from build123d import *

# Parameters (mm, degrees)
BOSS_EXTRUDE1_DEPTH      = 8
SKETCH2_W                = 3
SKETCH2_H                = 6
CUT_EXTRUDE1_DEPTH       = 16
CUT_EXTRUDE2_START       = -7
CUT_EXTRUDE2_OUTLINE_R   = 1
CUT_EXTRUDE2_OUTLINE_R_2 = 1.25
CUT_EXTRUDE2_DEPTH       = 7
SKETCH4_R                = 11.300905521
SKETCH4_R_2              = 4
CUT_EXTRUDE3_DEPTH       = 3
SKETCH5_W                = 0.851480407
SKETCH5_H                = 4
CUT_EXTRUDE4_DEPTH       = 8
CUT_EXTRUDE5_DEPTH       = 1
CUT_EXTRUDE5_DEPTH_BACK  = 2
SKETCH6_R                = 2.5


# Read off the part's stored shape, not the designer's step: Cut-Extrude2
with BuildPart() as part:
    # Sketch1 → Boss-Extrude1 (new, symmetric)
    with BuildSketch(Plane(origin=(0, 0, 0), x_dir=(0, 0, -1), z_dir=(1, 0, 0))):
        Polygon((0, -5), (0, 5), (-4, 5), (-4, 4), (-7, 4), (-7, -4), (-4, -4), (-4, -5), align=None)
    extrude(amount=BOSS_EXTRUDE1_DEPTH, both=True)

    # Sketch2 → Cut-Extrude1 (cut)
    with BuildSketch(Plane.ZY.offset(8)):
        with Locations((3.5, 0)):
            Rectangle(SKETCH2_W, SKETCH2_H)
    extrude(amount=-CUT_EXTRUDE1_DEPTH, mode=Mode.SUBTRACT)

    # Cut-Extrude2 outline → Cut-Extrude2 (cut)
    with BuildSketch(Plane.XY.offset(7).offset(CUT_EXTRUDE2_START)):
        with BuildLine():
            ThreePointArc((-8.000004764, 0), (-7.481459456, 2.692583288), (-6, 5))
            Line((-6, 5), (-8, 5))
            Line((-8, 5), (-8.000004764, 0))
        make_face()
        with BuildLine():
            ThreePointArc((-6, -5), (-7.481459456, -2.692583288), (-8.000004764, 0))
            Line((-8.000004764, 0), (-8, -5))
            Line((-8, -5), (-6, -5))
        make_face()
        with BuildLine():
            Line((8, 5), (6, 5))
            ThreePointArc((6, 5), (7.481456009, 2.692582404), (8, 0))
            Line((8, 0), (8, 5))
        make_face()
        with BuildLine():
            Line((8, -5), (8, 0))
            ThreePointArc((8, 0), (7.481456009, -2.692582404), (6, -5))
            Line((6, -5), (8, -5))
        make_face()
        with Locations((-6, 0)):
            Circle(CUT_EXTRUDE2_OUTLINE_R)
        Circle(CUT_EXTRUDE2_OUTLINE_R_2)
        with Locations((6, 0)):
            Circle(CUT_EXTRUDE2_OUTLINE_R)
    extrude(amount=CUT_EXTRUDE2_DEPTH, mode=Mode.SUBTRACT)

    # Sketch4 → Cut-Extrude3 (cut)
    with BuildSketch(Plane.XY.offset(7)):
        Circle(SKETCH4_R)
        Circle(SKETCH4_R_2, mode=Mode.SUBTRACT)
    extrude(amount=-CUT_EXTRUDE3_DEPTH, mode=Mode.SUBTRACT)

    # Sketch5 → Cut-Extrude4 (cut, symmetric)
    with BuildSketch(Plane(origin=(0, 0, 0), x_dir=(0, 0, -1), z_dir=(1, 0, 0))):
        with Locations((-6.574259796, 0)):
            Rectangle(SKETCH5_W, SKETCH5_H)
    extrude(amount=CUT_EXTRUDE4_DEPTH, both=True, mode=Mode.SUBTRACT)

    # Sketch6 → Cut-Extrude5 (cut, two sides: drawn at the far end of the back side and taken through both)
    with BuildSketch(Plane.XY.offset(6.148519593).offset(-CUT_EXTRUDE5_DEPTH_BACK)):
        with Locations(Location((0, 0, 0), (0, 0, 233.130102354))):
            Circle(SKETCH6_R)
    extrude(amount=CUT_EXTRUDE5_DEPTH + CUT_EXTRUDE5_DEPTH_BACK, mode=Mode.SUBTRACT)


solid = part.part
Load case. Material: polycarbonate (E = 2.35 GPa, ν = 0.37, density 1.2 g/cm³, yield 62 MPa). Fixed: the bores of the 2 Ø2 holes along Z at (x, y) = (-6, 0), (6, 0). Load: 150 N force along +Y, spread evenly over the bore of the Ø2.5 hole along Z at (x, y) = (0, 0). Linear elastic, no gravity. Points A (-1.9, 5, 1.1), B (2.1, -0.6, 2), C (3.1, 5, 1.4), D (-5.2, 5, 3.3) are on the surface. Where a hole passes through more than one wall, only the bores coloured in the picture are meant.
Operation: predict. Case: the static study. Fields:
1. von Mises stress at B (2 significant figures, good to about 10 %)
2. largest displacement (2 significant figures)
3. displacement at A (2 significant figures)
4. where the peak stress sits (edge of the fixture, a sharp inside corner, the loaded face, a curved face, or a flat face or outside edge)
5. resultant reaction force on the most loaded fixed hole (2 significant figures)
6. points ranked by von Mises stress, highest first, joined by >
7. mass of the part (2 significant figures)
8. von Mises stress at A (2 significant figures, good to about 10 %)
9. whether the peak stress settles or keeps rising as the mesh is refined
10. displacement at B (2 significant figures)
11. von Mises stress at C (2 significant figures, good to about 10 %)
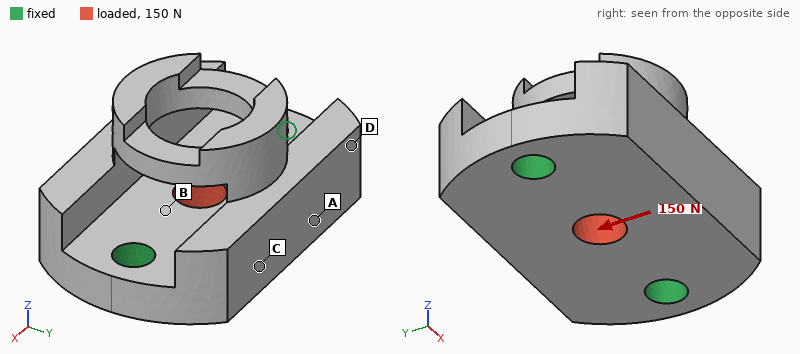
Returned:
9.4 MPa
37 µm
25 µm
edge of the fixture
75 N
B > A > C > D
0.53 g
7.3 MPa
keeps rising
27 µm
3.9 MPa
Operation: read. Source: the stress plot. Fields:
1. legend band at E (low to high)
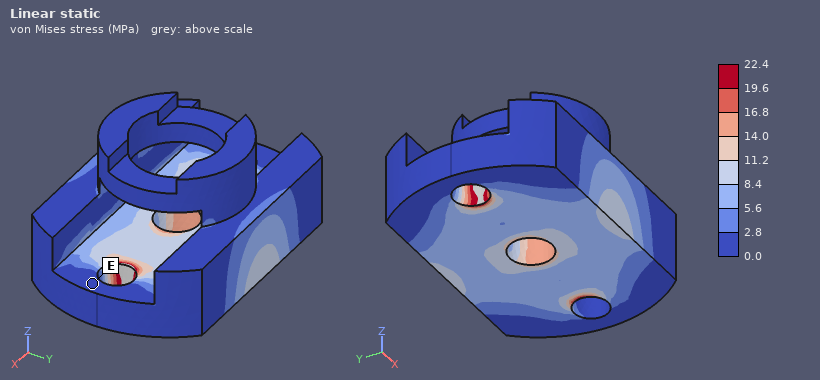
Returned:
0.0 to 2.8 MPa
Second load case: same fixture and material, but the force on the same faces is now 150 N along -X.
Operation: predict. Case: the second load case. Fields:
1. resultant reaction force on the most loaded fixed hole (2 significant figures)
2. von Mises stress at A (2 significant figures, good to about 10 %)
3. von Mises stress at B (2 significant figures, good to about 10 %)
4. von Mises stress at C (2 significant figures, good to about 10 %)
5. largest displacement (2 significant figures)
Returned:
75 N
1.4 MPa
10 MPa
1.4 MPa
19 µm
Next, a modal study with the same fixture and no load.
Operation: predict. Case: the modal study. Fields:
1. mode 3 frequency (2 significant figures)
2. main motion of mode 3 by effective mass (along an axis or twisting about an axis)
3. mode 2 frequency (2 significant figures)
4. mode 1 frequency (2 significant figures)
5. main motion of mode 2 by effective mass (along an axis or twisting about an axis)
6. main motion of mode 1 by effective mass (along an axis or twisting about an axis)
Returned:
15 kHz
along X
11 kHz
7400 Hz
along Z
along Y
